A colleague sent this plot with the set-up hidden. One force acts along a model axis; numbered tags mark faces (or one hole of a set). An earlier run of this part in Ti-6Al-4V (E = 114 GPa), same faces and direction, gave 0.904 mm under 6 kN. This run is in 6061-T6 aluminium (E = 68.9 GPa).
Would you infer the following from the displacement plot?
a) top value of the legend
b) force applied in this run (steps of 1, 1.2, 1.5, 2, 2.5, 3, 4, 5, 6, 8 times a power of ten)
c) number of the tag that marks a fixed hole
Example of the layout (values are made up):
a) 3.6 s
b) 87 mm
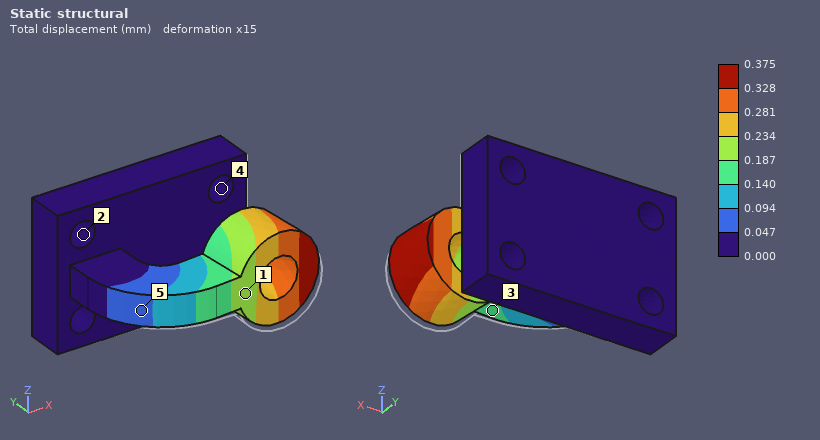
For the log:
a) 0.375 mm
b) 1.5 kN
c) 2
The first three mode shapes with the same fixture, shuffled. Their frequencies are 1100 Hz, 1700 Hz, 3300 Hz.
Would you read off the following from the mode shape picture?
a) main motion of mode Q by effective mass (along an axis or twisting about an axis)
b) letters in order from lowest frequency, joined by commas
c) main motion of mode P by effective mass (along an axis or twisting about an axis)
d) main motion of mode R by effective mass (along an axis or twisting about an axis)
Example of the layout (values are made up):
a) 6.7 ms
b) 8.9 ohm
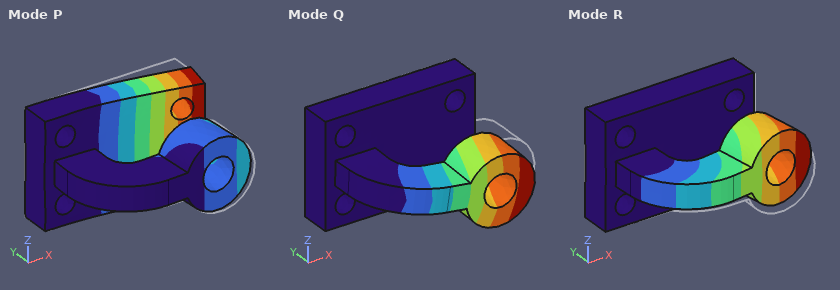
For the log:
a) along Z
b) Q, R, P
c) along Y
d) along Y
